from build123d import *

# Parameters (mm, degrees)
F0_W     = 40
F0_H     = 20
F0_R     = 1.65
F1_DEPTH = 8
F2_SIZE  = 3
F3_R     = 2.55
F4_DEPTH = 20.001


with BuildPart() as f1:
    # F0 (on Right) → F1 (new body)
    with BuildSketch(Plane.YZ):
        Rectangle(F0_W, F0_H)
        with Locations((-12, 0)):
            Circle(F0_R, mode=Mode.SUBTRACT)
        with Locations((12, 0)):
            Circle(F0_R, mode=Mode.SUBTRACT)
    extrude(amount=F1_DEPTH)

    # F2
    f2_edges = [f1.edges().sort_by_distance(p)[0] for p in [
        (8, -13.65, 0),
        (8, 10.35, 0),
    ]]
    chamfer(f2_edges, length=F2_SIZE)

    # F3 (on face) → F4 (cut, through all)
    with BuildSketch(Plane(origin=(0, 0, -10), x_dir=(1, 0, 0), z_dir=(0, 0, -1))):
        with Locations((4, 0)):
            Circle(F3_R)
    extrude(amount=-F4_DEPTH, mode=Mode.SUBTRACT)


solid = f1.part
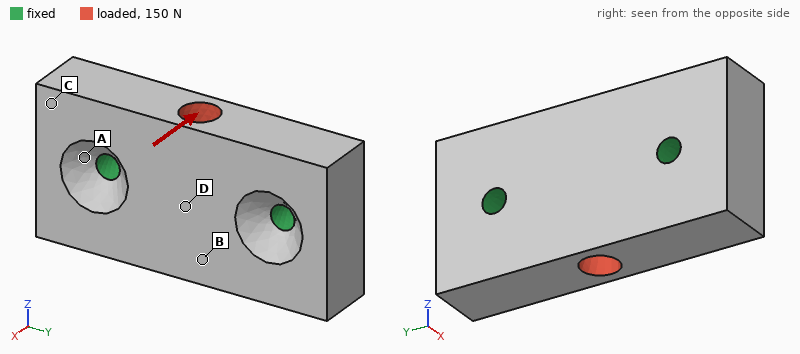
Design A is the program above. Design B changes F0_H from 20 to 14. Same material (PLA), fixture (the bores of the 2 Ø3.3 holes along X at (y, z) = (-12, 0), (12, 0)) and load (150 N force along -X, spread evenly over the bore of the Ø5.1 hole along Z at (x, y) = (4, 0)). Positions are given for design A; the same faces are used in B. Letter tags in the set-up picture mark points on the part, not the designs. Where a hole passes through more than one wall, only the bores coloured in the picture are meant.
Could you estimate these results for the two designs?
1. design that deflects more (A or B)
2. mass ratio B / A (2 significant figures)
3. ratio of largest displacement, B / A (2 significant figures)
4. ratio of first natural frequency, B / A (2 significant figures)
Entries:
B
0.68
1.1
1.6
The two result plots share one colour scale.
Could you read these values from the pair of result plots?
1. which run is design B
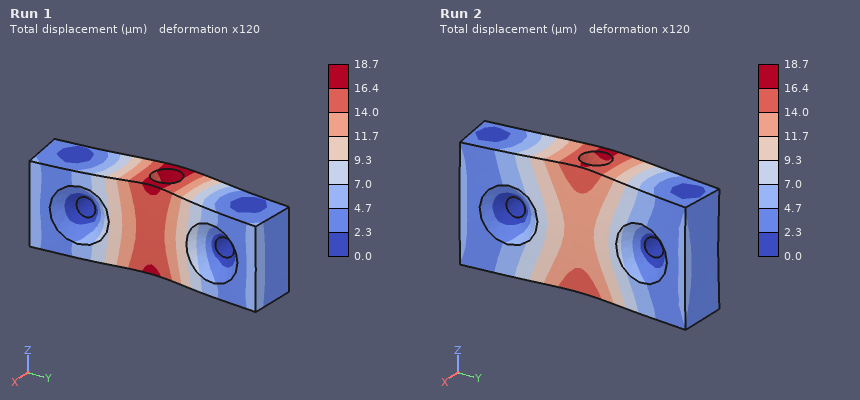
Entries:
Run 1
